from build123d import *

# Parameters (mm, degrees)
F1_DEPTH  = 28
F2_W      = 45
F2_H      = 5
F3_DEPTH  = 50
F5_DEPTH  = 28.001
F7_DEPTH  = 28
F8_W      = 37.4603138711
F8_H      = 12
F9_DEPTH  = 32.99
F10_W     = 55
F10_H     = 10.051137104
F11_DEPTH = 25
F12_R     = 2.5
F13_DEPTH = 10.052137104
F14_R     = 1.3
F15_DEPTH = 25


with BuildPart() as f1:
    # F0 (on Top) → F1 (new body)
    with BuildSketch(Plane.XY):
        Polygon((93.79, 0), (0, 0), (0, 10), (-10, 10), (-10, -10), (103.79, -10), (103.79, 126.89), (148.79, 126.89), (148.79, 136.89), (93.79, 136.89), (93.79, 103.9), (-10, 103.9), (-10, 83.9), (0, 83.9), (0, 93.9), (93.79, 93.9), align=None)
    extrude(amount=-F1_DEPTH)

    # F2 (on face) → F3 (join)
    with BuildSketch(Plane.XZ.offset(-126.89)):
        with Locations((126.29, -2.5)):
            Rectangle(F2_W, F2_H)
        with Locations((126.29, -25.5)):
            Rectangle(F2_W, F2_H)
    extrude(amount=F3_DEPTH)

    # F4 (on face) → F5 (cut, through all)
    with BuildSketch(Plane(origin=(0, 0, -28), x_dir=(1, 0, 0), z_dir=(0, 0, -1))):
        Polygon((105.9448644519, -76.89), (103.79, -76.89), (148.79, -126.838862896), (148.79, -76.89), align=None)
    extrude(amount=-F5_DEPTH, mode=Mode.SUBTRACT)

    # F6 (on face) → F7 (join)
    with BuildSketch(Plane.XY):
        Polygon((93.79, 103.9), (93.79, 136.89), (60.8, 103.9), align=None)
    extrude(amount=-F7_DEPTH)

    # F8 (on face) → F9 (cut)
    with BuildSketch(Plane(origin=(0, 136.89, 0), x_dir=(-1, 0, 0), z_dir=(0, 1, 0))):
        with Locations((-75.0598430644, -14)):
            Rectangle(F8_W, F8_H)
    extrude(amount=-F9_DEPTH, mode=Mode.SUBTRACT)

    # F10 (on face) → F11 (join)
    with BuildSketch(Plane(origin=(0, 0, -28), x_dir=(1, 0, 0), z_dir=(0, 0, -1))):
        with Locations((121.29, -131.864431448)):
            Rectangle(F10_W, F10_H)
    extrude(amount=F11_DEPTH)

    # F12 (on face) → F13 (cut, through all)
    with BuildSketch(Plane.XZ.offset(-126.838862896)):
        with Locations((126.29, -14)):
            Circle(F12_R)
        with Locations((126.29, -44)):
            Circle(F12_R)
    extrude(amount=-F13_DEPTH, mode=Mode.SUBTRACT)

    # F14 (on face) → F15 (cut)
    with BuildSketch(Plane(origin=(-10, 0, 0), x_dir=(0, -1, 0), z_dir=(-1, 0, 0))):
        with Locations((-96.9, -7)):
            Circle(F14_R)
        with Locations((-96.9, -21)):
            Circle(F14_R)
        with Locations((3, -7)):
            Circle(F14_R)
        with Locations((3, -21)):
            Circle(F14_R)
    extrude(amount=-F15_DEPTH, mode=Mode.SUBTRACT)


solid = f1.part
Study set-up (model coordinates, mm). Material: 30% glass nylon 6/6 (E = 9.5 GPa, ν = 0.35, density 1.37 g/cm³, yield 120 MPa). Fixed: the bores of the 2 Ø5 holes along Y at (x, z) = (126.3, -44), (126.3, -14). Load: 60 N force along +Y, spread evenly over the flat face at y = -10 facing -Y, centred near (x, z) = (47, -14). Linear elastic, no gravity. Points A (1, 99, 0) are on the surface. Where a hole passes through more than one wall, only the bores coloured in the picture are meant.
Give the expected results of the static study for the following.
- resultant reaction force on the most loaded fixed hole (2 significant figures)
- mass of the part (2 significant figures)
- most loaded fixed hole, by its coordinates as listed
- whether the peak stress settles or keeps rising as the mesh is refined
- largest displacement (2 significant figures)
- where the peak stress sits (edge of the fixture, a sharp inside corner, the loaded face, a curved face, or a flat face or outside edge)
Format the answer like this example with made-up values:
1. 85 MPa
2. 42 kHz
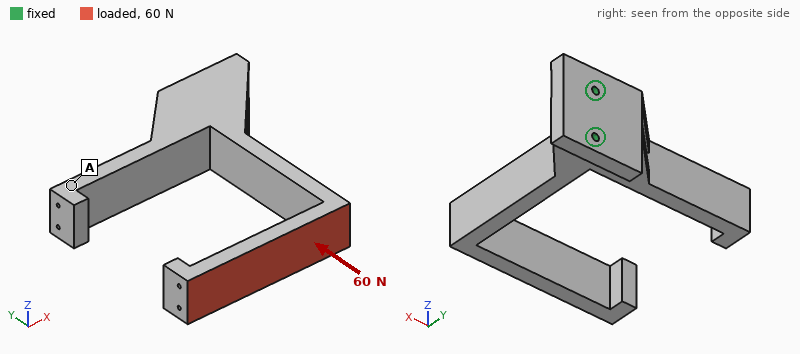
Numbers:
1. 55 N
2. 210 g
3. (126.3, -14)
4. keeps rising
5. 2.1 mm
6. edge of the fixture
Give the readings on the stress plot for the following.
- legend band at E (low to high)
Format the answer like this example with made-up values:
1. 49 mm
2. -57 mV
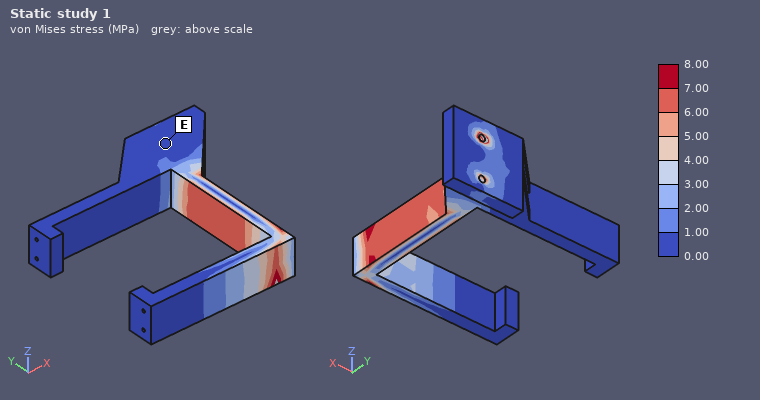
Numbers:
1. 0.00 to 1.00 MPa
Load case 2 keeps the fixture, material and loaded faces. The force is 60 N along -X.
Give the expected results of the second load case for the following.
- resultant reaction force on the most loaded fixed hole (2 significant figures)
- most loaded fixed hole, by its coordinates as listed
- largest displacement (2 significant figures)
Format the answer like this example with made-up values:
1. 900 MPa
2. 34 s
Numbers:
1. 60 N
2. (126.3, -14)
3. 2.0 mm
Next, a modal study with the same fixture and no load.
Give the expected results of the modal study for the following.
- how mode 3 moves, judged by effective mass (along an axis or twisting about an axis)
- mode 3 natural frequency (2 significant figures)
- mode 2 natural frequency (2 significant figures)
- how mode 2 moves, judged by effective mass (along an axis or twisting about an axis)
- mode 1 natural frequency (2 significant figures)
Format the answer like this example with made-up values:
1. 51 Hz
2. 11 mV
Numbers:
1. along X
2. 300 Hz
3. 170 Hz
4. along Z
5. 120 Hz
